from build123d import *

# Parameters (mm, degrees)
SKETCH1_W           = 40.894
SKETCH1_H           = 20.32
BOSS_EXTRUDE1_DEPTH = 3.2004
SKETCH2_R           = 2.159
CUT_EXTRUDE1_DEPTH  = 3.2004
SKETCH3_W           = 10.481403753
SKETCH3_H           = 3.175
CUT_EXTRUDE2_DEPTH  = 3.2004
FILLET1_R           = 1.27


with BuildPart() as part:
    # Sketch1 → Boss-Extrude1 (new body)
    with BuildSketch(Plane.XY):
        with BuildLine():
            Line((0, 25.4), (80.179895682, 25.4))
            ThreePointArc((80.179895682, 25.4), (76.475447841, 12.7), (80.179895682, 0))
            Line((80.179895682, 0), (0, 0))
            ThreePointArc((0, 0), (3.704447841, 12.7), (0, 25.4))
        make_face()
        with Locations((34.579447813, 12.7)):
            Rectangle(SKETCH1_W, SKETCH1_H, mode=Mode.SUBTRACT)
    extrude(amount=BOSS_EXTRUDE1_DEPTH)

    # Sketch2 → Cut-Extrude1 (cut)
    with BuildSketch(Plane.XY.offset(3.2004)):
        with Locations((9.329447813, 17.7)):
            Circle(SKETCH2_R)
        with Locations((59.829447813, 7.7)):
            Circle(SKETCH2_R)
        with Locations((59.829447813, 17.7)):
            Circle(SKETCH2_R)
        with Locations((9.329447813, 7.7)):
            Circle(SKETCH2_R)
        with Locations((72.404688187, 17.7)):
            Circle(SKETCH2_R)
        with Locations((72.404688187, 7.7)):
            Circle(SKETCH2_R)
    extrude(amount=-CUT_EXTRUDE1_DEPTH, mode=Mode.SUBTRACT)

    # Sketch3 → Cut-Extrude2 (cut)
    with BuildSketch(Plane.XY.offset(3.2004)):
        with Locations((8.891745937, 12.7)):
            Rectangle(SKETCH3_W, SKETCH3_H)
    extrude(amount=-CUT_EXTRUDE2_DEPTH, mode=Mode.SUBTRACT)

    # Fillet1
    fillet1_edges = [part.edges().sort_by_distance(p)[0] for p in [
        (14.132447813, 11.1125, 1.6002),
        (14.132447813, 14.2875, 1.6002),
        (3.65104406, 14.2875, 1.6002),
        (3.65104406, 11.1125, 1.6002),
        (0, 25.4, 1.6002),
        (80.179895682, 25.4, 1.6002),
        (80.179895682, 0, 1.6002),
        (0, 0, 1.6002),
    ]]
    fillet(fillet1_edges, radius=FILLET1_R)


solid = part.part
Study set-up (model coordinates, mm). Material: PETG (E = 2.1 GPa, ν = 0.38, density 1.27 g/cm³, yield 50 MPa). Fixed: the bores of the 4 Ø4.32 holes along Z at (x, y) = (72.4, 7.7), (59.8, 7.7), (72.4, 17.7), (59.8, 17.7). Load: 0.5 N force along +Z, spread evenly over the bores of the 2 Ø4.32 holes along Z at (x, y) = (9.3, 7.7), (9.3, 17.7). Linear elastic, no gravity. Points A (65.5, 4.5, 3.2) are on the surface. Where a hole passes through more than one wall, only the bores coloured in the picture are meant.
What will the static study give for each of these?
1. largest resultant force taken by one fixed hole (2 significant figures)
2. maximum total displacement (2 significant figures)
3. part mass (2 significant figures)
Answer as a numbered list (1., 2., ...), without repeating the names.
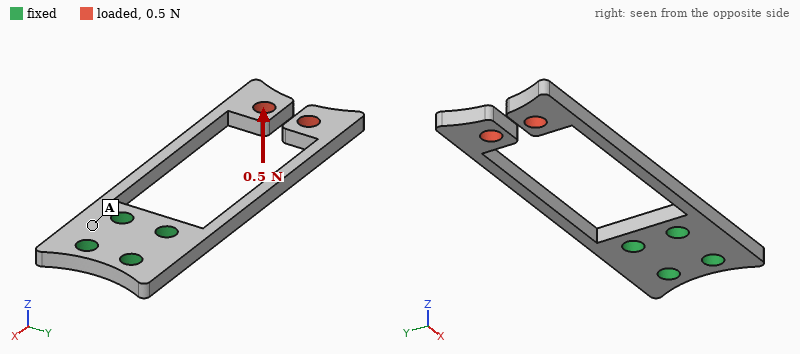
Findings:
1. 0.53 N
2. 0.88 mm
3. 3.9 g
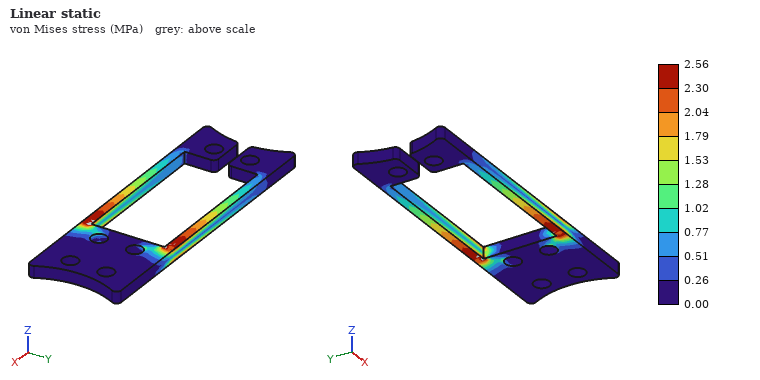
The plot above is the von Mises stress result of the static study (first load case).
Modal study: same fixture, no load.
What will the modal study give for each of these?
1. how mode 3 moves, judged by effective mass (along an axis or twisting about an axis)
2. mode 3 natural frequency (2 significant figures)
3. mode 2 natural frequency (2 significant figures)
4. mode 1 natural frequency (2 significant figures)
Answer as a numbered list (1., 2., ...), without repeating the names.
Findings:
1. along Z
2. 130 Hz
3. 110 Hz
4. 110 Hz
